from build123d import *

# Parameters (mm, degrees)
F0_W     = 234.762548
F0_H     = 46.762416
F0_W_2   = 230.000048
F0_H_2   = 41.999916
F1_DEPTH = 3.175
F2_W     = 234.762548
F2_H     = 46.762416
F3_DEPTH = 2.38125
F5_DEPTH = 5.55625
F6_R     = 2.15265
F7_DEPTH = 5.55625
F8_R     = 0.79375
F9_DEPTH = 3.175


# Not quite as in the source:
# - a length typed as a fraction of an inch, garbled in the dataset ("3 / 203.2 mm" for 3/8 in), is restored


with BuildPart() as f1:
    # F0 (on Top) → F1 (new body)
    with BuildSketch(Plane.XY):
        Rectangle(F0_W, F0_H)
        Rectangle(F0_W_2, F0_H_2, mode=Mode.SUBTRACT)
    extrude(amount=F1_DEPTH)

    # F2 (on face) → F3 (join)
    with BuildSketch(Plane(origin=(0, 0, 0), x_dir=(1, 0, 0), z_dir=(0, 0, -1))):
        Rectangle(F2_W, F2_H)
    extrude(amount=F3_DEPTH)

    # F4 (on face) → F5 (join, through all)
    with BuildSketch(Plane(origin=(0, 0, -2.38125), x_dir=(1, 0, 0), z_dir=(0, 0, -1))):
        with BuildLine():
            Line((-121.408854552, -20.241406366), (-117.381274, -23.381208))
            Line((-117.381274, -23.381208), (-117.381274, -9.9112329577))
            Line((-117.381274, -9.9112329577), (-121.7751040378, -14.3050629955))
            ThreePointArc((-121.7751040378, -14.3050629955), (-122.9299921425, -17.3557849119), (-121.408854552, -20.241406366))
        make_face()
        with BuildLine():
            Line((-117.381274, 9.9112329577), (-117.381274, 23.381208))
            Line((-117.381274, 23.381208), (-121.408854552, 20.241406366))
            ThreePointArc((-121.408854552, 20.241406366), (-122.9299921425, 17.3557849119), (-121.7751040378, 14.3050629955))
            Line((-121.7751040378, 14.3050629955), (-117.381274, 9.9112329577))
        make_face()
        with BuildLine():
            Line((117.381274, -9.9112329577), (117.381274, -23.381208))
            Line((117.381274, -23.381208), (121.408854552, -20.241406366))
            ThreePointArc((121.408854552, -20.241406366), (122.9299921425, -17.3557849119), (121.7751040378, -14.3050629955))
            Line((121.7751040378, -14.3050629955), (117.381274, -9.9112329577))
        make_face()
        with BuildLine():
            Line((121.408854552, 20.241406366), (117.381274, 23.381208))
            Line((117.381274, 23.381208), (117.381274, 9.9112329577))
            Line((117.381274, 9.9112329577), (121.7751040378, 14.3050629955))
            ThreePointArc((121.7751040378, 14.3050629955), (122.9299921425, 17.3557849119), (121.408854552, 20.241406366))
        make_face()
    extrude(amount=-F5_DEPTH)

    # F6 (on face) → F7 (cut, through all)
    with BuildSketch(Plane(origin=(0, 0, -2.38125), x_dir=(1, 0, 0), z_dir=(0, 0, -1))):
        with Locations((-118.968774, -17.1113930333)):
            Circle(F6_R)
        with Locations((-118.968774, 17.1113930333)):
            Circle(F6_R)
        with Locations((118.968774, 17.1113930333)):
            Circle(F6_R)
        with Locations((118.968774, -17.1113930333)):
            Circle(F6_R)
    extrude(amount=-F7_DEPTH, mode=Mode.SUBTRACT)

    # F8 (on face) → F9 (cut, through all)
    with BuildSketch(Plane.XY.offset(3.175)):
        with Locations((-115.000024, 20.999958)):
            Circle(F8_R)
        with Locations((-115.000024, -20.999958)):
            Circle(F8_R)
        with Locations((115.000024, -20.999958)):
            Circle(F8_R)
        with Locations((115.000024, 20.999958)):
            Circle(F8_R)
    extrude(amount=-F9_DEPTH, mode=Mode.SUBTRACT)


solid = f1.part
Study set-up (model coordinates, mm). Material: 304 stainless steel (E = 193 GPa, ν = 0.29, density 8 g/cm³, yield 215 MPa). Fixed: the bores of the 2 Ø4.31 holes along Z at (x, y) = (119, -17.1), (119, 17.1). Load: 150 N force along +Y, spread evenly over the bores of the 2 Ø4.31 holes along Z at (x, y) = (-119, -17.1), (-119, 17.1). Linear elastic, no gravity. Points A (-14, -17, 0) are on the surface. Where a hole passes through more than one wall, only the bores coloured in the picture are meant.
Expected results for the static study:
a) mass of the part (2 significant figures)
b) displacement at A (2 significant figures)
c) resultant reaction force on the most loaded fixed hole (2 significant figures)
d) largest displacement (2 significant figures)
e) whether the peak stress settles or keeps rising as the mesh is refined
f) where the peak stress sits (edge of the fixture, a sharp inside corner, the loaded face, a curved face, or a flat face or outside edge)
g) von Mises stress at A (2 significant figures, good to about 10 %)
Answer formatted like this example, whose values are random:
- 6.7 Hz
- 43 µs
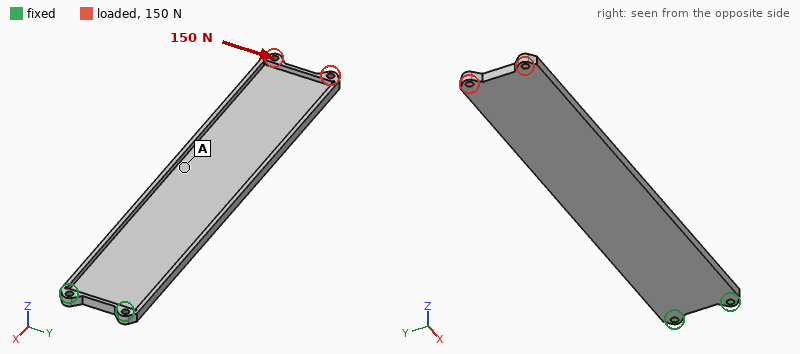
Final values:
- 250 g
- 0.067 mm
- 990 N
- 0.18 mm
- keeps rising
- edge of the fixture
- 12 MPa
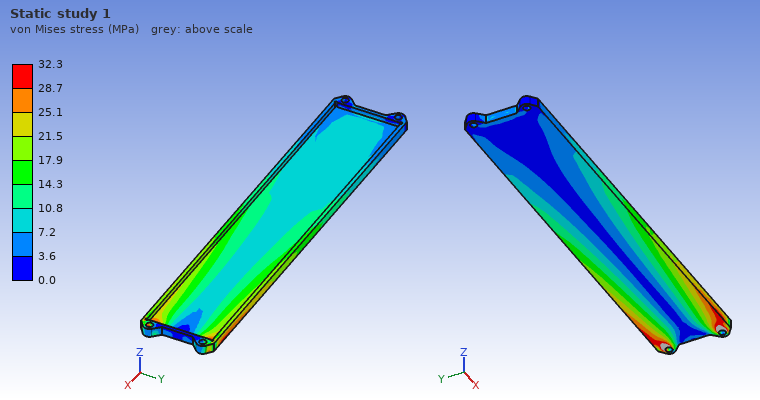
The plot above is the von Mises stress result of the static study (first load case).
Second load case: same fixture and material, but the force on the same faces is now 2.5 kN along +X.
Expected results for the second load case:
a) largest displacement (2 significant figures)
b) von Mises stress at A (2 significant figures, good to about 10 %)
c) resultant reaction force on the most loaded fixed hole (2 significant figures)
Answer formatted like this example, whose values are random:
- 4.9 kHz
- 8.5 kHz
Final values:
- 2.8 mm
- 36 MPa
- 1.3 kN
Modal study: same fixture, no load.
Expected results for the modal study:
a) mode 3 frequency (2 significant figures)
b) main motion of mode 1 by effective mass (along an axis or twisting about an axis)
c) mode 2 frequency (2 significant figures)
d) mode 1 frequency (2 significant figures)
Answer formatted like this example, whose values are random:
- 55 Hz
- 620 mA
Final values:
- 340 Hz
- along Z
- 330 Hz
- 53 Hz
